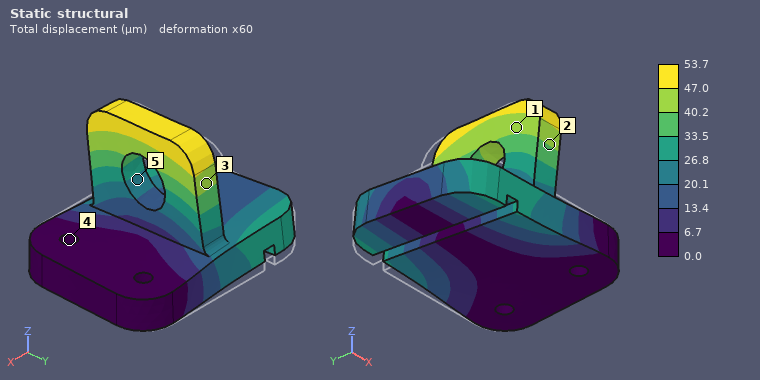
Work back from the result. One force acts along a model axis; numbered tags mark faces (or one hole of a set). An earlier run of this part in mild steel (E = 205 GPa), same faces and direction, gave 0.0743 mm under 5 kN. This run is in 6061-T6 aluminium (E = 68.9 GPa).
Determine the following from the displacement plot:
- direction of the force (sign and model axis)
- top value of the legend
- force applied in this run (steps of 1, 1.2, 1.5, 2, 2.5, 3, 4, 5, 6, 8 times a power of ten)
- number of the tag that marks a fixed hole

-Y
53.7 µm
1.2 kN
4
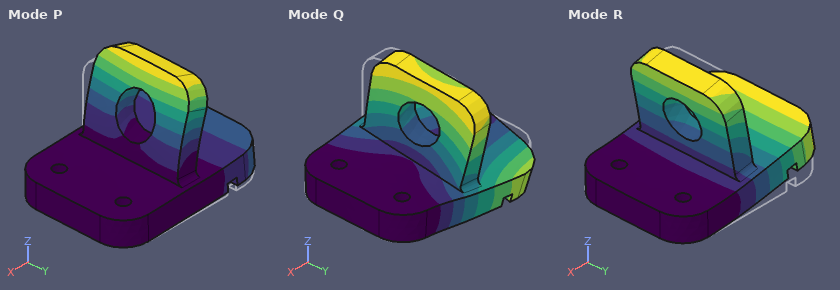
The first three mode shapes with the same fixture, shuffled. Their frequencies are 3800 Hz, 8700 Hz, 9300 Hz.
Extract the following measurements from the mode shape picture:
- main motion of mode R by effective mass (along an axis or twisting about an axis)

along Z
